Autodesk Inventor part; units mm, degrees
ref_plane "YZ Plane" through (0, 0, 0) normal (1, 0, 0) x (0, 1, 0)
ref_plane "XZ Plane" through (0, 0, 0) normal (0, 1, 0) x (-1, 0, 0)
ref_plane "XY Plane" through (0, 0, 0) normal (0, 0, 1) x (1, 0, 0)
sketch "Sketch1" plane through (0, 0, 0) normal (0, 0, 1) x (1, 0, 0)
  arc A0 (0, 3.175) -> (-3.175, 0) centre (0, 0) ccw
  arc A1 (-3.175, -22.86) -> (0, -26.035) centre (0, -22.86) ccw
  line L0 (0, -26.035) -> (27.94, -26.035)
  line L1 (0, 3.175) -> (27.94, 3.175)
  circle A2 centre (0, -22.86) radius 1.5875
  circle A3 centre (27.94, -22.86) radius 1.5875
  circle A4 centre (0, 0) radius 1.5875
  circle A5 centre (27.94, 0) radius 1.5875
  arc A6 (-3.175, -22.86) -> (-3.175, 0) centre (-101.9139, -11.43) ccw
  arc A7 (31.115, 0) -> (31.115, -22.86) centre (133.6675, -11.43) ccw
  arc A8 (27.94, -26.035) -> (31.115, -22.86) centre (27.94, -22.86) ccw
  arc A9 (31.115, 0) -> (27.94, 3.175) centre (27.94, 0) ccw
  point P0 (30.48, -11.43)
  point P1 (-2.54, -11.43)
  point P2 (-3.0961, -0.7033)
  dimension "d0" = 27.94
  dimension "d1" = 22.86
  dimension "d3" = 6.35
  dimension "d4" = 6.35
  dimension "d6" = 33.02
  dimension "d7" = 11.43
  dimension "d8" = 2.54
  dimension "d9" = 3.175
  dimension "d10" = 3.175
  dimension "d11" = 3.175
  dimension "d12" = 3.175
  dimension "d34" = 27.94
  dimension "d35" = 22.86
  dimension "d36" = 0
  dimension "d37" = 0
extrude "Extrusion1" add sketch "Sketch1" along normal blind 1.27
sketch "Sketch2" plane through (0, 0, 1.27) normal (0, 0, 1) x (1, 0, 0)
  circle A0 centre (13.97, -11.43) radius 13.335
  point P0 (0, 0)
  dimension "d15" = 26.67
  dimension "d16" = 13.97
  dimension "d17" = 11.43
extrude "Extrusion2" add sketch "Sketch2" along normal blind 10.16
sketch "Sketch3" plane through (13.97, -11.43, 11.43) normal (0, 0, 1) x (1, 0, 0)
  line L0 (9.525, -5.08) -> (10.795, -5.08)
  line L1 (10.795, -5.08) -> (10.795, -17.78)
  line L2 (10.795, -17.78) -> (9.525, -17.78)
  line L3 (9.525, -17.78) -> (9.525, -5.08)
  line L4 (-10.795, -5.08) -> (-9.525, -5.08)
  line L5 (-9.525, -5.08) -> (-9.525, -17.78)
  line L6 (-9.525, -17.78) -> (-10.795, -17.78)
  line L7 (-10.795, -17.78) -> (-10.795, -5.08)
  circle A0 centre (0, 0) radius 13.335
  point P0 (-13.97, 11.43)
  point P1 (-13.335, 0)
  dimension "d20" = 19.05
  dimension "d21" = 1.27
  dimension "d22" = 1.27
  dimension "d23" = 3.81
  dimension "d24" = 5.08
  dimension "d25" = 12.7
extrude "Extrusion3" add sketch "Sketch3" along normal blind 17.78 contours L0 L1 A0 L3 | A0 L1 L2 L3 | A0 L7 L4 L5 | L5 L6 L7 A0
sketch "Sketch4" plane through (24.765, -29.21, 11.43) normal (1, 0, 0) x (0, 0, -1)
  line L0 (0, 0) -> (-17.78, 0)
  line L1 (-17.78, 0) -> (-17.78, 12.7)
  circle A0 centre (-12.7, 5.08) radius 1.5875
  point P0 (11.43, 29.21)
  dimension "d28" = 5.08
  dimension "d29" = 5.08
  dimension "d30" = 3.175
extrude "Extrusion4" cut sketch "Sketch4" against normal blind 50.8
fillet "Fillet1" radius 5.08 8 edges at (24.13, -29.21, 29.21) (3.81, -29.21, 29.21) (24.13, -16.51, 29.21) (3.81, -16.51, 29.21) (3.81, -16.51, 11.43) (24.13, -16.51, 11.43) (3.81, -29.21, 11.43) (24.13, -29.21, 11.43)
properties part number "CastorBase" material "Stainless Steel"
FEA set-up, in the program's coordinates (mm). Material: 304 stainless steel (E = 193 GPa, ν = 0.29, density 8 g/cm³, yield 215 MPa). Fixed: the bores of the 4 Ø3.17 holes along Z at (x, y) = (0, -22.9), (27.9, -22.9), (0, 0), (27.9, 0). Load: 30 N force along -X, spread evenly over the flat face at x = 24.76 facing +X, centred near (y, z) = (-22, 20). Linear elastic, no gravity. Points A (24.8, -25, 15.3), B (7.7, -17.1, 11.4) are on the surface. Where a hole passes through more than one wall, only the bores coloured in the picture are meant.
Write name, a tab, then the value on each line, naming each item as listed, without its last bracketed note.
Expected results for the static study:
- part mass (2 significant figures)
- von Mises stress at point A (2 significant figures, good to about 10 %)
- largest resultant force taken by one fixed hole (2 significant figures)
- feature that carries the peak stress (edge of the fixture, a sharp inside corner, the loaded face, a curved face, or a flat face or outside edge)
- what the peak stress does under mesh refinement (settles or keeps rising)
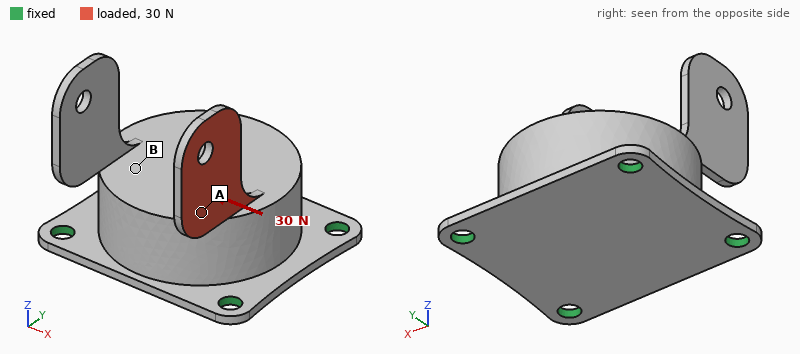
part mass	59 g
von Mises stress at point A	26 MPa
largest resultant force taken by one fixed hole	17 N
feature that carries the peak stress	a sharp inside corner
what the peak stress does under mesh refinement	keeps rising
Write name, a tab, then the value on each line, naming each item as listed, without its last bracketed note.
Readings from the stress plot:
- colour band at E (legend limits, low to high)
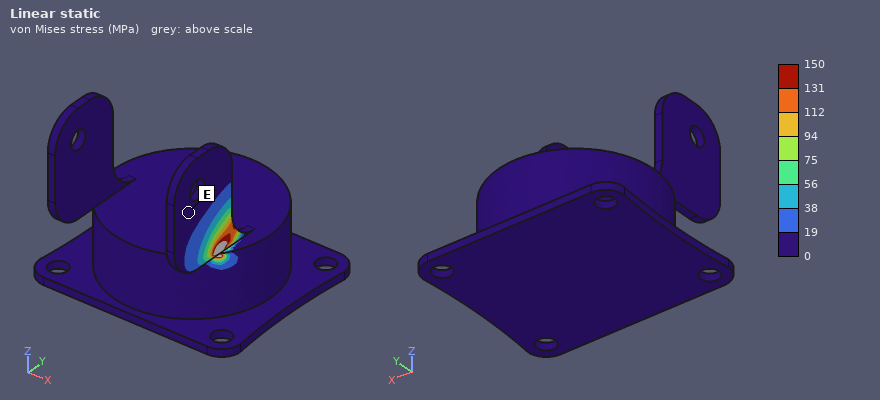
colour band at E	0 to 19 MPa
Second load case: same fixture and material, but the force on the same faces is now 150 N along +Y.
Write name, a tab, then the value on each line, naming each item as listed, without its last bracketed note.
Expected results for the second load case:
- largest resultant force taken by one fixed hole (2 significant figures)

largest resultant force taken by one fixed hole	92 N
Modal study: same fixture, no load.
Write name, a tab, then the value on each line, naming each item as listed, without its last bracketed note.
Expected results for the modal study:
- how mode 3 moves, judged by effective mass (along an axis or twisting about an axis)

how mode 3 moves, judged by effective mass	along Y
